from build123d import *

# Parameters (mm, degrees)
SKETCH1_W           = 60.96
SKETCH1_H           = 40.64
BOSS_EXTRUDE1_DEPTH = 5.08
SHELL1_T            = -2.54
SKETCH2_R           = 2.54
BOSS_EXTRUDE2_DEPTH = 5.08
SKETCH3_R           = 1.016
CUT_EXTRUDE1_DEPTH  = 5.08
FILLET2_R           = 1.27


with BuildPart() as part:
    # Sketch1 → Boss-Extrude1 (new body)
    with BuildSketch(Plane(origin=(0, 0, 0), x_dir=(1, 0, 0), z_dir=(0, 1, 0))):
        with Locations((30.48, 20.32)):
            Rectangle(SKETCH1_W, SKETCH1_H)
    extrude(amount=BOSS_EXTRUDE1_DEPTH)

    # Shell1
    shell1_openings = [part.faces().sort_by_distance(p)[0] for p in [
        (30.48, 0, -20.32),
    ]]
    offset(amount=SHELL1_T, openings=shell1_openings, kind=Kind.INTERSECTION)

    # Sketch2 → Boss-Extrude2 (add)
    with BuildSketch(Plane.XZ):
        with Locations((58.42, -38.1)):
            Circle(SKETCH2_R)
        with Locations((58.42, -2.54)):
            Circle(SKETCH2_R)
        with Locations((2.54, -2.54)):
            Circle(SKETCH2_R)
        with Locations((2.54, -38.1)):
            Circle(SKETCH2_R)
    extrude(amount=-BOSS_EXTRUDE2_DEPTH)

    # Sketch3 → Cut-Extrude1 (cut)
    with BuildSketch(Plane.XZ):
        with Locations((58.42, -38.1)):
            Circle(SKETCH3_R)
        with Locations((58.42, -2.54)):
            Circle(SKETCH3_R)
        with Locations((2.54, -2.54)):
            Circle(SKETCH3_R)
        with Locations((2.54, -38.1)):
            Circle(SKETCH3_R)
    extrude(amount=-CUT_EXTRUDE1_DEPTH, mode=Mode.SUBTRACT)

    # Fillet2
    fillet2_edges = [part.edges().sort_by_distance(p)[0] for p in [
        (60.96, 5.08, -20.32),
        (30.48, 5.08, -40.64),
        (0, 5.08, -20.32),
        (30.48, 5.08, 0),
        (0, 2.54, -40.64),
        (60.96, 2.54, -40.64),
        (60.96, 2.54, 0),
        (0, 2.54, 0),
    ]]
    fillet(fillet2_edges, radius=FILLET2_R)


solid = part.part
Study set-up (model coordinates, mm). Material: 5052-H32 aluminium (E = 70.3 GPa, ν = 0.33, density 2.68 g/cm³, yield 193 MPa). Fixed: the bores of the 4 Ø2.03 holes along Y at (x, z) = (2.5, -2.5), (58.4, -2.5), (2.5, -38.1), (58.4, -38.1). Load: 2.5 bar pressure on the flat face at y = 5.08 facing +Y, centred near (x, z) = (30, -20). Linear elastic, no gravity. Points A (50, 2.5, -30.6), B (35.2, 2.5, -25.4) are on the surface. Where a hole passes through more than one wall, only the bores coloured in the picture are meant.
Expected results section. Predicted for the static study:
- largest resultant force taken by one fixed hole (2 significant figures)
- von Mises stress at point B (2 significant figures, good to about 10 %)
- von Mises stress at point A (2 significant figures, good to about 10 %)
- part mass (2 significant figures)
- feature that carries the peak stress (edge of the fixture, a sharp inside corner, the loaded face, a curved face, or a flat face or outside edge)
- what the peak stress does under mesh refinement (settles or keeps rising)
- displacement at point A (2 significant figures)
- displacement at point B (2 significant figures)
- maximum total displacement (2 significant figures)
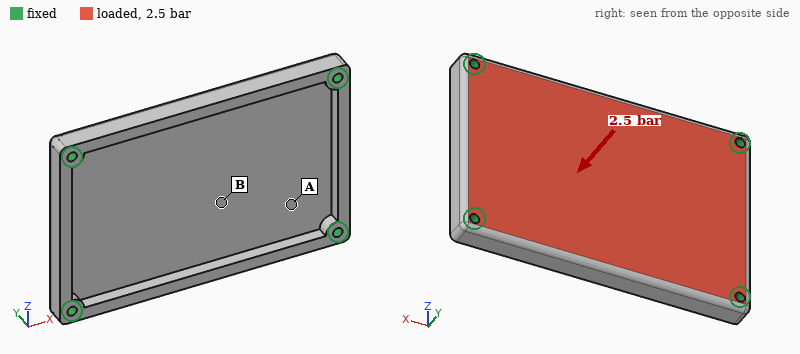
160 N
18 MPa
7.6 MPa
20 g
edge of the fixture
keeps rising
19 µm
49 µm
53 µm
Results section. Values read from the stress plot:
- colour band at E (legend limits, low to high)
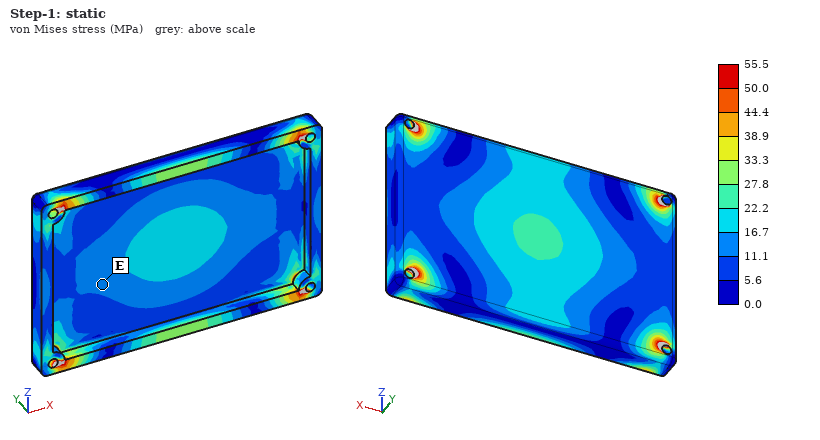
11.1 to 16.7 MPa
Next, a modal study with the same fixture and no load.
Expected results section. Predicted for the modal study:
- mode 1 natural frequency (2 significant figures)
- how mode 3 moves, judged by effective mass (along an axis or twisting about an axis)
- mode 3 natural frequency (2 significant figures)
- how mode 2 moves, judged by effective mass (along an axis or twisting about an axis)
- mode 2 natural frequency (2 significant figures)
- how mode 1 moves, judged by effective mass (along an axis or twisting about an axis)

4900 Hz
twisting about Z
11 kHz
twisting about X
7800 Hz
along Y
